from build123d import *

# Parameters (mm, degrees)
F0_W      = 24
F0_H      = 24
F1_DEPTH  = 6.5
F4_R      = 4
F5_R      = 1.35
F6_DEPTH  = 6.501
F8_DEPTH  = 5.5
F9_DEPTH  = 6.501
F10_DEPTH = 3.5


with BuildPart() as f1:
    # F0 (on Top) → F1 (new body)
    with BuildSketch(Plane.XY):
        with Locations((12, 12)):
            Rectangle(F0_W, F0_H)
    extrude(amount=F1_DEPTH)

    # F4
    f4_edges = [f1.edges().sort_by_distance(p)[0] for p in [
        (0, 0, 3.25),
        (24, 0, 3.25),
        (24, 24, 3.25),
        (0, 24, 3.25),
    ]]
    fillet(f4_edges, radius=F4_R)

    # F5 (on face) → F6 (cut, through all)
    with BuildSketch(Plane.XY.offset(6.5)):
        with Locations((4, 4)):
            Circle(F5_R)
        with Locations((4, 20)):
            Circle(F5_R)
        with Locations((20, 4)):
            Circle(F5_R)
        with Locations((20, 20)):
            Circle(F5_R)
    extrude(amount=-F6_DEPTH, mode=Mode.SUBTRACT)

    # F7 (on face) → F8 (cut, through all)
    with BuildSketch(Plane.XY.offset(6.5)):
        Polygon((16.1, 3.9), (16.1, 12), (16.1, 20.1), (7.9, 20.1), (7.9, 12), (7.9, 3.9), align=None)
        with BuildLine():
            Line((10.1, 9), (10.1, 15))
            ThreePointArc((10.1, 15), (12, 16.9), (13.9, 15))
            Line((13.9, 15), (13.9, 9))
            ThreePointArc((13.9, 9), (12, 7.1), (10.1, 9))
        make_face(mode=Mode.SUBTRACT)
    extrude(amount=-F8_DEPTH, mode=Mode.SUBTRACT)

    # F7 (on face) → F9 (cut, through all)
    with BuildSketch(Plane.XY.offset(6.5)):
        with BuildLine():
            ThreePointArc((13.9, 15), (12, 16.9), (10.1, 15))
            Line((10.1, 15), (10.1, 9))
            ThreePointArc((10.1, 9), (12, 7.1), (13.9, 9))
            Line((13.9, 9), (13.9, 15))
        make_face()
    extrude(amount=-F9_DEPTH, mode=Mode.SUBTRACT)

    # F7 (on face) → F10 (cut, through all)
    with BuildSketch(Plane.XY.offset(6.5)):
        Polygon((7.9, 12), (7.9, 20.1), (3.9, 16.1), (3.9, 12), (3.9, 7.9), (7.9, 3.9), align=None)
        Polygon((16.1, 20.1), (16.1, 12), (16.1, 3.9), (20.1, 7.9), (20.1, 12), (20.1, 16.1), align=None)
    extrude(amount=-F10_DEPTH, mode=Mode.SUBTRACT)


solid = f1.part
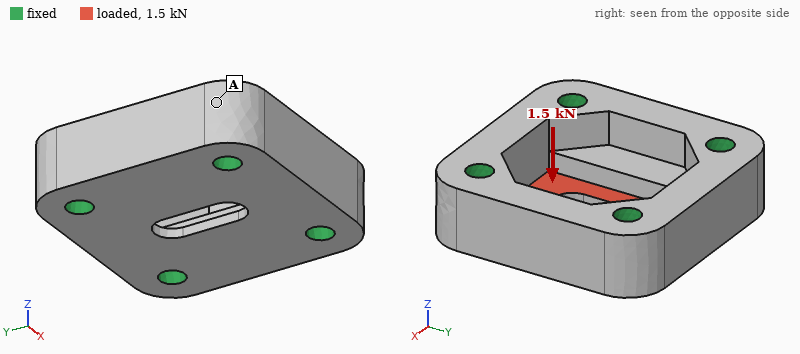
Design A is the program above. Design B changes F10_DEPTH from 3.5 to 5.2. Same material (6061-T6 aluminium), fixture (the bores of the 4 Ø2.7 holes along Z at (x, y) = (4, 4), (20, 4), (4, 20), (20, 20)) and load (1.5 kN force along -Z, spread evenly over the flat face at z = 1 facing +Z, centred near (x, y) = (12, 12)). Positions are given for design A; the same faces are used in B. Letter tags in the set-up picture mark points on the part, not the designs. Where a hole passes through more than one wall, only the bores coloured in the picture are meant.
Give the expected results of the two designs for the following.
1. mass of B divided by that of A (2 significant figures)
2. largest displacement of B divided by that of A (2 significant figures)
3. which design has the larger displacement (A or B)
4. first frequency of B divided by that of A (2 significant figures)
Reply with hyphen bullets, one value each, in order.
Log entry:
- 0.93
- 3.2
- B
- 0.63
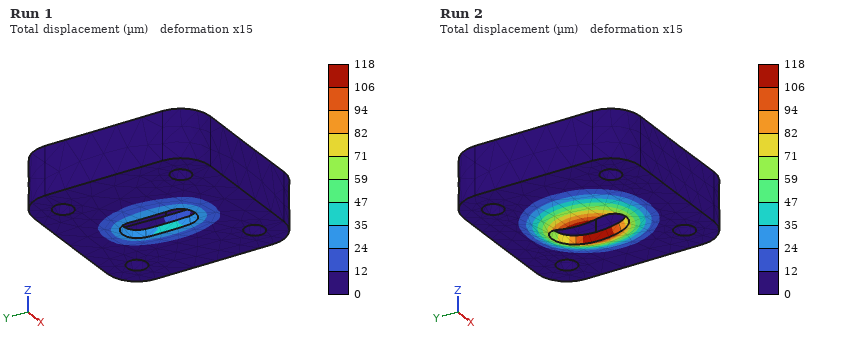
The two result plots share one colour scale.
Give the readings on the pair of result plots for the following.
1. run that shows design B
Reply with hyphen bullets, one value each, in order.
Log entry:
- Run 2
